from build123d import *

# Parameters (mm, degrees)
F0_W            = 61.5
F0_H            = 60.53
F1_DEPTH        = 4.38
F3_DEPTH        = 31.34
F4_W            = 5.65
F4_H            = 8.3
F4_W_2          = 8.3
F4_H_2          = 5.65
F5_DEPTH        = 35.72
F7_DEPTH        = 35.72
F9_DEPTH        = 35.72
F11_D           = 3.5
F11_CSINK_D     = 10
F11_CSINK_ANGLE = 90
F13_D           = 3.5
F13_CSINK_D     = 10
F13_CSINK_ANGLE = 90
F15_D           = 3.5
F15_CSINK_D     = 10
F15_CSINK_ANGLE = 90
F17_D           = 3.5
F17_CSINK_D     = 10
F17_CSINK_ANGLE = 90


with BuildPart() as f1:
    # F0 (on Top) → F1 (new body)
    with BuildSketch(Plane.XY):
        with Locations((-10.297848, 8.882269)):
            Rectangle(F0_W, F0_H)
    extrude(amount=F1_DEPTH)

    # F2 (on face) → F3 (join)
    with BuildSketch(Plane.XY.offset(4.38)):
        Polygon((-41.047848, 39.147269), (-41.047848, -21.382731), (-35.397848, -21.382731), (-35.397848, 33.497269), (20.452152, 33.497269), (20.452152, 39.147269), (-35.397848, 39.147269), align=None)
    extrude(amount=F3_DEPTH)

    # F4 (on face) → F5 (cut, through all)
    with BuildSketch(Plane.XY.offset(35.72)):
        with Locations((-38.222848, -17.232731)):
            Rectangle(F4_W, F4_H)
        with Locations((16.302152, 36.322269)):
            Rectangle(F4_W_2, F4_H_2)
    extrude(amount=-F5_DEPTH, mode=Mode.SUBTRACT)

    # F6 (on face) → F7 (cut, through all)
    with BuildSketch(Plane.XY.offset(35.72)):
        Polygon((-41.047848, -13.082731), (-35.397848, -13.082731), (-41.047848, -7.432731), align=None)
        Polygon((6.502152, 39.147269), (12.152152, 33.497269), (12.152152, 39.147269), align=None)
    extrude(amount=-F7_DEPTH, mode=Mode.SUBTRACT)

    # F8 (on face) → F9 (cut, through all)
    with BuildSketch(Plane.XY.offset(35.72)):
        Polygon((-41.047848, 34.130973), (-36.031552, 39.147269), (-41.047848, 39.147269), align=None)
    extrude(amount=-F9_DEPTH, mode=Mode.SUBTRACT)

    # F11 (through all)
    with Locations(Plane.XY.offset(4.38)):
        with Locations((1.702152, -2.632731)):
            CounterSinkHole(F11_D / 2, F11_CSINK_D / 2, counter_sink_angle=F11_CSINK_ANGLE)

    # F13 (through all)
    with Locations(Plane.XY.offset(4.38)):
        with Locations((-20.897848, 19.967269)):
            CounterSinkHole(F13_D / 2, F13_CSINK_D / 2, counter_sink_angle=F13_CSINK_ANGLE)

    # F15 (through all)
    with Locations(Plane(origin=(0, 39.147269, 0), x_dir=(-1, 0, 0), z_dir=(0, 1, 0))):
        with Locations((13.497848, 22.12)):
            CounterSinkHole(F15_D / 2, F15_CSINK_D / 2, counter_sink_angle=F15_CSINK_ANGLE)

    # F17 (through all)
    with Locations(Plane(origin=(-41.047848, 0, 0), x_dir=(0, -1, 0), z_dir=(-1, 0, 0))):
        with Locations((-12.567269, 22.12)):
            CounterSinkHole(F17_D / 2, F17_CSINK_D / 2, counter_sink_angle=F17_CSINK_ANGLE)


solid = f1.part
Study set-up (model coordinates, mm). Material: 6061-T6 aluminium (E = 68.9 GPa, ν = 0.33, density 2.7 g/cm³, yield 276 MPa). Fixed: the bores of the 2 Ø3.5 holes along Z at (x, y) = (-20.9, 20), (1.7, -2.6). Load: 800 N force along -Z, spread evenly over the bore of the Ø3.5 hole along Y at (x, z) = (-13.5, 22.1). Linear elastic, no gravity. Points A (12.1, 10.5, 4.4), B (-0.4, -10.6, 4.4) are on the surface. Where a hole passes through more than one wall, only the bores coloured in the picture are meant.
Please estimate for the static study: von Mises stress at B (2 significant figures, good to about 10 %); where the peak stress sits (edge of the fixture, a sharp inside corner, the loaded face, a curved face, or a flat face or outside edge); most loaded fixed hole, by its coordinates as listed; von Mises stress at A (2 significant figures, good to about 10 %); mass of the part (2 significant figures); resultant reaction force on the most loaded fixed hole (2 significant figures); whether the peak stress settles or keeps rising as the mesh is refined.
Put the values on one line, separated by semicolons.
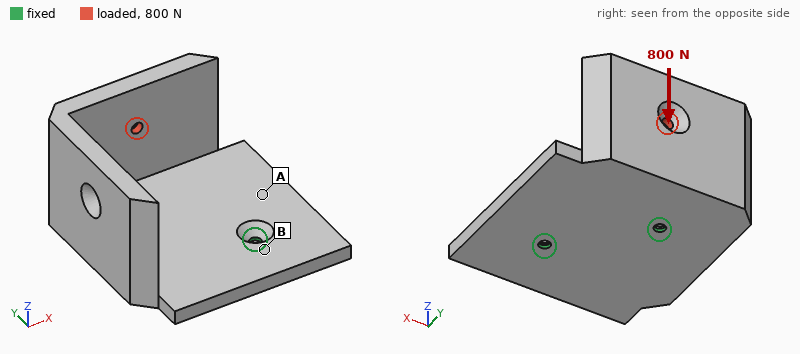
44 MPa; edge of the fixture; (-20.9, 20); 21 MPa; 85 g; 940 N; keeps rising
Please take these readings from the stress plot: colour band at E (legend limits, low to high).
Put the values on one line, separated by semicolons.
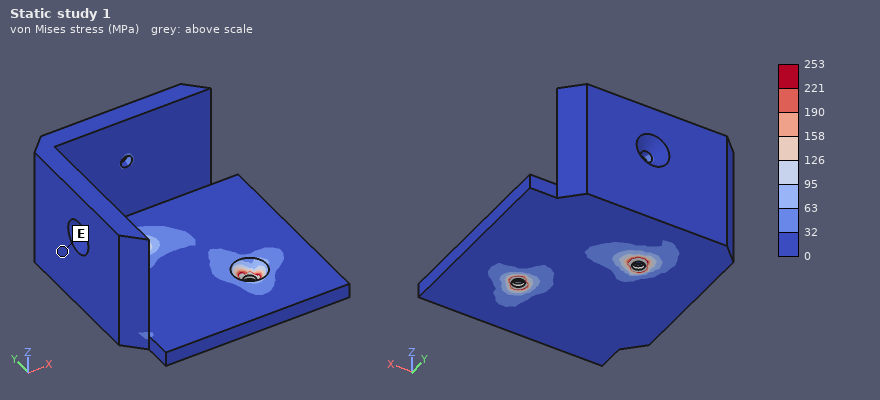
0 to 32 MPa
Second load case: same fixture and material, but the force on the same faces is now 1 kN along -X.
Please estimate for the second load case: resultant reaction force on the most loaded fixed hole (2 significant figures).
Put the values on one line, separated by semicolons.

1.2 kN
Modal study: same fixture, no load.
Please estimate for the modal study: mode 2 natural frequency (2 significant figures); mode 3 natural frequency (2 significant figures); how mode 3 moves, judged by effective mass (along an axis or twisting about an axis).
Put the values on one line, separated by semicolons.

1700 Hz; 3500 Hz; along Z
